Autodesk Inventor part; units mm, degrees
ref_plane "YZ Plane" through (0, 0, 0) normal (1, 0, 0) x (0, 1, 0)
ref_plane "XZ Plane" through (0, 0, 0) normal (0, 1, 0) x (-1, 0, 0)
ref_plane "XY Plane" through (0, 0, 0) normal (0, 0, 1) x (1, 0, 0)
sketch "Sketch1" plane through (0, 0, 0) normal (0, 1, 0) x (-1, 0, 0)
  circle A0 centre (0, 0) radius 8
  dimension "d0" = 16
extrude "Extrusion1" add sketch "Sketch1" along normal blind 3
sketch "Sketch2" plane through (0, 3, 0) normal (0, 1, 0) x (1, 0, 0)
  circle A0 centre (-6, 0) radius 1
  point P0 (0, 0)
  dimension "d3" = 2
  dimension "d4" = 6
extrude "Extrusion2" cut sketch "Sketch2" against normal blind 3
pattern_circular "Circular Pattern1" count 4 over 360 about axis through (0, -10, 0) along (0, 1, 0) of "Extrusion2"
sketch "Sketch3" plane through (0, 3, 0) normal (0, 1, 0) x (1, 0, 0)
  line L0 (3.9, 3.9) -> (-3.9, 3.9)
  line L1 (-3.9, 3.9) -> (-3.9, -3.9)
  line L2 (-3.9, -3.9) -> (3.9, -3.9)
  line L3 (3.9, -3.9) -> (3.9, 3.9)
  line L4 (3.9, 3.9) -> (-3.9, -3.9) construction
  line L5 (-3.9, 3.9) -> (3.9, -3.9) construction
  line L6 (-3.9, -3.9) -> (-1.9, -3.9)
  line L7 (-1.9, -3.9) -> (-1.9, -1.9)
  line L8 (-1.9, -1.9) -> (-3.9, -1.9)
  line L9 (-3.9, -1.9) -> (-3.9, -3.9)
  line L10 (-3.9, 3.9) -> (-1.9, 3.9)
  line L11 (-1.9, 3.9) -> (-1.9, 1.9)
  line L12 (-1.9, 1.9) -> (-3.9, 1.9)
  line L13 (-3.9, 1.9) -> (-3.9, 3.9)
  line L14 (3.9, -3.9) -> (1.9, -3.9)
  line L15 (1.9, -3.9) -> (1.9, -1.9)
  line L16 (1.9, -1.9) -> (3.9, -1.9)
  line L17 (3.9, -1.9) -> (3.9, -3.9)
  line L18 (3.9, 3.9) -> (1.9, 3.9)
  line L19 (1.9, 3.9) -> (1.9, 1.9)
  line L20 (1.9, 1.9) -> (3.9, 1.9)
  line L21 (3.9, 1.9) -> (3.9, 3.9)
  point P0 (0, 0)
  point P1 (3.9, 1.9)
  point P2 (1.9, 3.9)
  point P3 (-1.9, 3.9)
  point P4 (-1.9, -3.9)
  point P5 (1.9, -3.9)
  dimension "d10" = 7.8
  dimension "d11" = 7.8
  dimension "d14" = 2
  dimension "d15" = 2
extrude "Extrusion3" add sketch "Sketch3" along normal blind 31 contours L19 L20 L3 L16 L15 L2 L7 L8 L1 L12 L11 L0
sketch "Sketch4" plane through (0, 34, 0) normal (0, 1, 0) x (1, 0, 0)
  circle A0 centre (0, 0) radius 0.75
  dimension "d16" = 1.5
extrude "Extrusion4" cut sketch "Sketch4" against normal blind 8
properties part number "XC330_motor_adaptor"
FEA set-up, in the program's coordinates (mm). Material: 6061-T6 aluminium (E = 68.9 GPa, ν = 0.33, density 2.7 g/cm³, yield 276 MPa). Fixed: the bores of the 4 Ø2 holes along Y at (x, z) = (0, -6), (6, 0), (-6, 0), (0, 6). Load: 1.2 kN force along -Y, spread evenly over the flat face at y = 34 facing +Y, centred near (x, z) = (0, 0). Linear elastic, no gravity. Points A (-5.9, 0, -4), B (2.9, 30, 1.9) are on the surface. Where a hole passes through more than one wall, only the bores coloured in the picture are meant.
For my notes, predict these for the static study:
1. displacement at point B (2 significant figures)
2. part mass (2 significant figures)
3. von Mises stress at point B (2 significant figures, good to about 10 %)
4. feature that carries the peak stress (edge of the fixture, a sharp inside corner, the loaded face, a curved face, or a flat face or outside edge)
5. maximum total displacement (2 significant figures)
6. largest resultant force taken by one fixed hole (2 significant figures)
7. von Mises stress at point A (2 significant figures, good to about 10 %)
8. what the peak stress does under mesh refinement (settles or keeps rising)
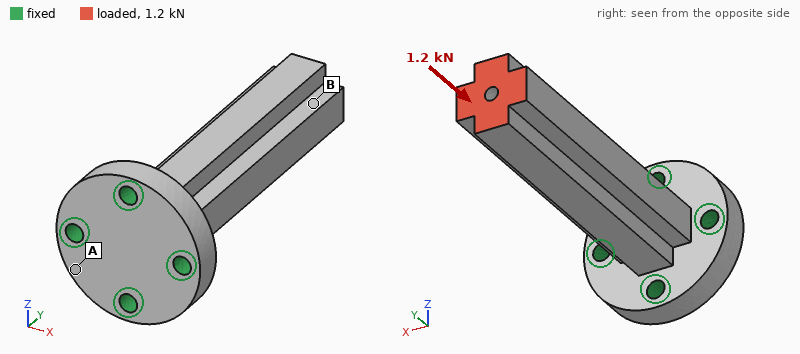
13 µm
5.2 g
28 MPa
edge of the fixture
15 µm
310 N
10 MPa
keeps rising
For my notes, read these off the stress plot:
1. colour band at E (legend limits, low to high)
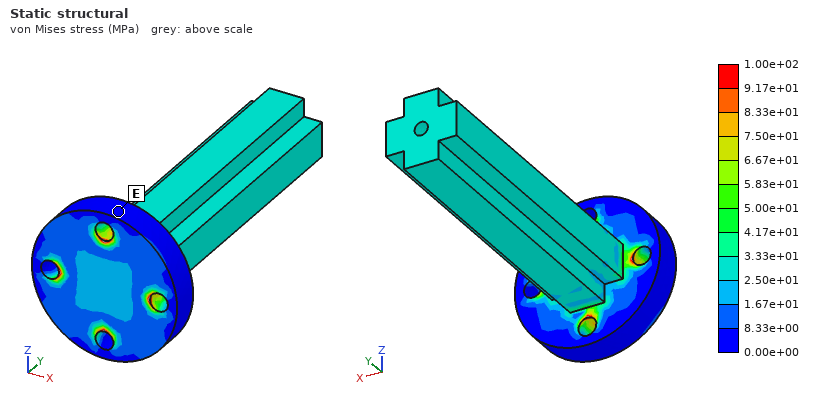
0.00e+00 to 8.33e+00 MPa
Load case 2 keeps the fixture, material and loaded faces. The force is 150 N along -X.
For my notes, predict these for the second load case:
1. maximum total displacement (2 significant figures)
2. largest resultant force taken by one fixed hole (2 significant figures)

0.16 mm
440 N
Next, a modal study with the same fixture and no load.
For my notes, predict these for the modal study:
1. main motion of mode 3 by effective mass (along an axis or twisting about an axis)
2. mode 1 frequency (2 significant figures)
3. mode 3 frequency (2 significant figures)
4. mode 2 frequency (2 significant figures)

twisting about Y
4900 Hz
21 kHz
4900 Hz
